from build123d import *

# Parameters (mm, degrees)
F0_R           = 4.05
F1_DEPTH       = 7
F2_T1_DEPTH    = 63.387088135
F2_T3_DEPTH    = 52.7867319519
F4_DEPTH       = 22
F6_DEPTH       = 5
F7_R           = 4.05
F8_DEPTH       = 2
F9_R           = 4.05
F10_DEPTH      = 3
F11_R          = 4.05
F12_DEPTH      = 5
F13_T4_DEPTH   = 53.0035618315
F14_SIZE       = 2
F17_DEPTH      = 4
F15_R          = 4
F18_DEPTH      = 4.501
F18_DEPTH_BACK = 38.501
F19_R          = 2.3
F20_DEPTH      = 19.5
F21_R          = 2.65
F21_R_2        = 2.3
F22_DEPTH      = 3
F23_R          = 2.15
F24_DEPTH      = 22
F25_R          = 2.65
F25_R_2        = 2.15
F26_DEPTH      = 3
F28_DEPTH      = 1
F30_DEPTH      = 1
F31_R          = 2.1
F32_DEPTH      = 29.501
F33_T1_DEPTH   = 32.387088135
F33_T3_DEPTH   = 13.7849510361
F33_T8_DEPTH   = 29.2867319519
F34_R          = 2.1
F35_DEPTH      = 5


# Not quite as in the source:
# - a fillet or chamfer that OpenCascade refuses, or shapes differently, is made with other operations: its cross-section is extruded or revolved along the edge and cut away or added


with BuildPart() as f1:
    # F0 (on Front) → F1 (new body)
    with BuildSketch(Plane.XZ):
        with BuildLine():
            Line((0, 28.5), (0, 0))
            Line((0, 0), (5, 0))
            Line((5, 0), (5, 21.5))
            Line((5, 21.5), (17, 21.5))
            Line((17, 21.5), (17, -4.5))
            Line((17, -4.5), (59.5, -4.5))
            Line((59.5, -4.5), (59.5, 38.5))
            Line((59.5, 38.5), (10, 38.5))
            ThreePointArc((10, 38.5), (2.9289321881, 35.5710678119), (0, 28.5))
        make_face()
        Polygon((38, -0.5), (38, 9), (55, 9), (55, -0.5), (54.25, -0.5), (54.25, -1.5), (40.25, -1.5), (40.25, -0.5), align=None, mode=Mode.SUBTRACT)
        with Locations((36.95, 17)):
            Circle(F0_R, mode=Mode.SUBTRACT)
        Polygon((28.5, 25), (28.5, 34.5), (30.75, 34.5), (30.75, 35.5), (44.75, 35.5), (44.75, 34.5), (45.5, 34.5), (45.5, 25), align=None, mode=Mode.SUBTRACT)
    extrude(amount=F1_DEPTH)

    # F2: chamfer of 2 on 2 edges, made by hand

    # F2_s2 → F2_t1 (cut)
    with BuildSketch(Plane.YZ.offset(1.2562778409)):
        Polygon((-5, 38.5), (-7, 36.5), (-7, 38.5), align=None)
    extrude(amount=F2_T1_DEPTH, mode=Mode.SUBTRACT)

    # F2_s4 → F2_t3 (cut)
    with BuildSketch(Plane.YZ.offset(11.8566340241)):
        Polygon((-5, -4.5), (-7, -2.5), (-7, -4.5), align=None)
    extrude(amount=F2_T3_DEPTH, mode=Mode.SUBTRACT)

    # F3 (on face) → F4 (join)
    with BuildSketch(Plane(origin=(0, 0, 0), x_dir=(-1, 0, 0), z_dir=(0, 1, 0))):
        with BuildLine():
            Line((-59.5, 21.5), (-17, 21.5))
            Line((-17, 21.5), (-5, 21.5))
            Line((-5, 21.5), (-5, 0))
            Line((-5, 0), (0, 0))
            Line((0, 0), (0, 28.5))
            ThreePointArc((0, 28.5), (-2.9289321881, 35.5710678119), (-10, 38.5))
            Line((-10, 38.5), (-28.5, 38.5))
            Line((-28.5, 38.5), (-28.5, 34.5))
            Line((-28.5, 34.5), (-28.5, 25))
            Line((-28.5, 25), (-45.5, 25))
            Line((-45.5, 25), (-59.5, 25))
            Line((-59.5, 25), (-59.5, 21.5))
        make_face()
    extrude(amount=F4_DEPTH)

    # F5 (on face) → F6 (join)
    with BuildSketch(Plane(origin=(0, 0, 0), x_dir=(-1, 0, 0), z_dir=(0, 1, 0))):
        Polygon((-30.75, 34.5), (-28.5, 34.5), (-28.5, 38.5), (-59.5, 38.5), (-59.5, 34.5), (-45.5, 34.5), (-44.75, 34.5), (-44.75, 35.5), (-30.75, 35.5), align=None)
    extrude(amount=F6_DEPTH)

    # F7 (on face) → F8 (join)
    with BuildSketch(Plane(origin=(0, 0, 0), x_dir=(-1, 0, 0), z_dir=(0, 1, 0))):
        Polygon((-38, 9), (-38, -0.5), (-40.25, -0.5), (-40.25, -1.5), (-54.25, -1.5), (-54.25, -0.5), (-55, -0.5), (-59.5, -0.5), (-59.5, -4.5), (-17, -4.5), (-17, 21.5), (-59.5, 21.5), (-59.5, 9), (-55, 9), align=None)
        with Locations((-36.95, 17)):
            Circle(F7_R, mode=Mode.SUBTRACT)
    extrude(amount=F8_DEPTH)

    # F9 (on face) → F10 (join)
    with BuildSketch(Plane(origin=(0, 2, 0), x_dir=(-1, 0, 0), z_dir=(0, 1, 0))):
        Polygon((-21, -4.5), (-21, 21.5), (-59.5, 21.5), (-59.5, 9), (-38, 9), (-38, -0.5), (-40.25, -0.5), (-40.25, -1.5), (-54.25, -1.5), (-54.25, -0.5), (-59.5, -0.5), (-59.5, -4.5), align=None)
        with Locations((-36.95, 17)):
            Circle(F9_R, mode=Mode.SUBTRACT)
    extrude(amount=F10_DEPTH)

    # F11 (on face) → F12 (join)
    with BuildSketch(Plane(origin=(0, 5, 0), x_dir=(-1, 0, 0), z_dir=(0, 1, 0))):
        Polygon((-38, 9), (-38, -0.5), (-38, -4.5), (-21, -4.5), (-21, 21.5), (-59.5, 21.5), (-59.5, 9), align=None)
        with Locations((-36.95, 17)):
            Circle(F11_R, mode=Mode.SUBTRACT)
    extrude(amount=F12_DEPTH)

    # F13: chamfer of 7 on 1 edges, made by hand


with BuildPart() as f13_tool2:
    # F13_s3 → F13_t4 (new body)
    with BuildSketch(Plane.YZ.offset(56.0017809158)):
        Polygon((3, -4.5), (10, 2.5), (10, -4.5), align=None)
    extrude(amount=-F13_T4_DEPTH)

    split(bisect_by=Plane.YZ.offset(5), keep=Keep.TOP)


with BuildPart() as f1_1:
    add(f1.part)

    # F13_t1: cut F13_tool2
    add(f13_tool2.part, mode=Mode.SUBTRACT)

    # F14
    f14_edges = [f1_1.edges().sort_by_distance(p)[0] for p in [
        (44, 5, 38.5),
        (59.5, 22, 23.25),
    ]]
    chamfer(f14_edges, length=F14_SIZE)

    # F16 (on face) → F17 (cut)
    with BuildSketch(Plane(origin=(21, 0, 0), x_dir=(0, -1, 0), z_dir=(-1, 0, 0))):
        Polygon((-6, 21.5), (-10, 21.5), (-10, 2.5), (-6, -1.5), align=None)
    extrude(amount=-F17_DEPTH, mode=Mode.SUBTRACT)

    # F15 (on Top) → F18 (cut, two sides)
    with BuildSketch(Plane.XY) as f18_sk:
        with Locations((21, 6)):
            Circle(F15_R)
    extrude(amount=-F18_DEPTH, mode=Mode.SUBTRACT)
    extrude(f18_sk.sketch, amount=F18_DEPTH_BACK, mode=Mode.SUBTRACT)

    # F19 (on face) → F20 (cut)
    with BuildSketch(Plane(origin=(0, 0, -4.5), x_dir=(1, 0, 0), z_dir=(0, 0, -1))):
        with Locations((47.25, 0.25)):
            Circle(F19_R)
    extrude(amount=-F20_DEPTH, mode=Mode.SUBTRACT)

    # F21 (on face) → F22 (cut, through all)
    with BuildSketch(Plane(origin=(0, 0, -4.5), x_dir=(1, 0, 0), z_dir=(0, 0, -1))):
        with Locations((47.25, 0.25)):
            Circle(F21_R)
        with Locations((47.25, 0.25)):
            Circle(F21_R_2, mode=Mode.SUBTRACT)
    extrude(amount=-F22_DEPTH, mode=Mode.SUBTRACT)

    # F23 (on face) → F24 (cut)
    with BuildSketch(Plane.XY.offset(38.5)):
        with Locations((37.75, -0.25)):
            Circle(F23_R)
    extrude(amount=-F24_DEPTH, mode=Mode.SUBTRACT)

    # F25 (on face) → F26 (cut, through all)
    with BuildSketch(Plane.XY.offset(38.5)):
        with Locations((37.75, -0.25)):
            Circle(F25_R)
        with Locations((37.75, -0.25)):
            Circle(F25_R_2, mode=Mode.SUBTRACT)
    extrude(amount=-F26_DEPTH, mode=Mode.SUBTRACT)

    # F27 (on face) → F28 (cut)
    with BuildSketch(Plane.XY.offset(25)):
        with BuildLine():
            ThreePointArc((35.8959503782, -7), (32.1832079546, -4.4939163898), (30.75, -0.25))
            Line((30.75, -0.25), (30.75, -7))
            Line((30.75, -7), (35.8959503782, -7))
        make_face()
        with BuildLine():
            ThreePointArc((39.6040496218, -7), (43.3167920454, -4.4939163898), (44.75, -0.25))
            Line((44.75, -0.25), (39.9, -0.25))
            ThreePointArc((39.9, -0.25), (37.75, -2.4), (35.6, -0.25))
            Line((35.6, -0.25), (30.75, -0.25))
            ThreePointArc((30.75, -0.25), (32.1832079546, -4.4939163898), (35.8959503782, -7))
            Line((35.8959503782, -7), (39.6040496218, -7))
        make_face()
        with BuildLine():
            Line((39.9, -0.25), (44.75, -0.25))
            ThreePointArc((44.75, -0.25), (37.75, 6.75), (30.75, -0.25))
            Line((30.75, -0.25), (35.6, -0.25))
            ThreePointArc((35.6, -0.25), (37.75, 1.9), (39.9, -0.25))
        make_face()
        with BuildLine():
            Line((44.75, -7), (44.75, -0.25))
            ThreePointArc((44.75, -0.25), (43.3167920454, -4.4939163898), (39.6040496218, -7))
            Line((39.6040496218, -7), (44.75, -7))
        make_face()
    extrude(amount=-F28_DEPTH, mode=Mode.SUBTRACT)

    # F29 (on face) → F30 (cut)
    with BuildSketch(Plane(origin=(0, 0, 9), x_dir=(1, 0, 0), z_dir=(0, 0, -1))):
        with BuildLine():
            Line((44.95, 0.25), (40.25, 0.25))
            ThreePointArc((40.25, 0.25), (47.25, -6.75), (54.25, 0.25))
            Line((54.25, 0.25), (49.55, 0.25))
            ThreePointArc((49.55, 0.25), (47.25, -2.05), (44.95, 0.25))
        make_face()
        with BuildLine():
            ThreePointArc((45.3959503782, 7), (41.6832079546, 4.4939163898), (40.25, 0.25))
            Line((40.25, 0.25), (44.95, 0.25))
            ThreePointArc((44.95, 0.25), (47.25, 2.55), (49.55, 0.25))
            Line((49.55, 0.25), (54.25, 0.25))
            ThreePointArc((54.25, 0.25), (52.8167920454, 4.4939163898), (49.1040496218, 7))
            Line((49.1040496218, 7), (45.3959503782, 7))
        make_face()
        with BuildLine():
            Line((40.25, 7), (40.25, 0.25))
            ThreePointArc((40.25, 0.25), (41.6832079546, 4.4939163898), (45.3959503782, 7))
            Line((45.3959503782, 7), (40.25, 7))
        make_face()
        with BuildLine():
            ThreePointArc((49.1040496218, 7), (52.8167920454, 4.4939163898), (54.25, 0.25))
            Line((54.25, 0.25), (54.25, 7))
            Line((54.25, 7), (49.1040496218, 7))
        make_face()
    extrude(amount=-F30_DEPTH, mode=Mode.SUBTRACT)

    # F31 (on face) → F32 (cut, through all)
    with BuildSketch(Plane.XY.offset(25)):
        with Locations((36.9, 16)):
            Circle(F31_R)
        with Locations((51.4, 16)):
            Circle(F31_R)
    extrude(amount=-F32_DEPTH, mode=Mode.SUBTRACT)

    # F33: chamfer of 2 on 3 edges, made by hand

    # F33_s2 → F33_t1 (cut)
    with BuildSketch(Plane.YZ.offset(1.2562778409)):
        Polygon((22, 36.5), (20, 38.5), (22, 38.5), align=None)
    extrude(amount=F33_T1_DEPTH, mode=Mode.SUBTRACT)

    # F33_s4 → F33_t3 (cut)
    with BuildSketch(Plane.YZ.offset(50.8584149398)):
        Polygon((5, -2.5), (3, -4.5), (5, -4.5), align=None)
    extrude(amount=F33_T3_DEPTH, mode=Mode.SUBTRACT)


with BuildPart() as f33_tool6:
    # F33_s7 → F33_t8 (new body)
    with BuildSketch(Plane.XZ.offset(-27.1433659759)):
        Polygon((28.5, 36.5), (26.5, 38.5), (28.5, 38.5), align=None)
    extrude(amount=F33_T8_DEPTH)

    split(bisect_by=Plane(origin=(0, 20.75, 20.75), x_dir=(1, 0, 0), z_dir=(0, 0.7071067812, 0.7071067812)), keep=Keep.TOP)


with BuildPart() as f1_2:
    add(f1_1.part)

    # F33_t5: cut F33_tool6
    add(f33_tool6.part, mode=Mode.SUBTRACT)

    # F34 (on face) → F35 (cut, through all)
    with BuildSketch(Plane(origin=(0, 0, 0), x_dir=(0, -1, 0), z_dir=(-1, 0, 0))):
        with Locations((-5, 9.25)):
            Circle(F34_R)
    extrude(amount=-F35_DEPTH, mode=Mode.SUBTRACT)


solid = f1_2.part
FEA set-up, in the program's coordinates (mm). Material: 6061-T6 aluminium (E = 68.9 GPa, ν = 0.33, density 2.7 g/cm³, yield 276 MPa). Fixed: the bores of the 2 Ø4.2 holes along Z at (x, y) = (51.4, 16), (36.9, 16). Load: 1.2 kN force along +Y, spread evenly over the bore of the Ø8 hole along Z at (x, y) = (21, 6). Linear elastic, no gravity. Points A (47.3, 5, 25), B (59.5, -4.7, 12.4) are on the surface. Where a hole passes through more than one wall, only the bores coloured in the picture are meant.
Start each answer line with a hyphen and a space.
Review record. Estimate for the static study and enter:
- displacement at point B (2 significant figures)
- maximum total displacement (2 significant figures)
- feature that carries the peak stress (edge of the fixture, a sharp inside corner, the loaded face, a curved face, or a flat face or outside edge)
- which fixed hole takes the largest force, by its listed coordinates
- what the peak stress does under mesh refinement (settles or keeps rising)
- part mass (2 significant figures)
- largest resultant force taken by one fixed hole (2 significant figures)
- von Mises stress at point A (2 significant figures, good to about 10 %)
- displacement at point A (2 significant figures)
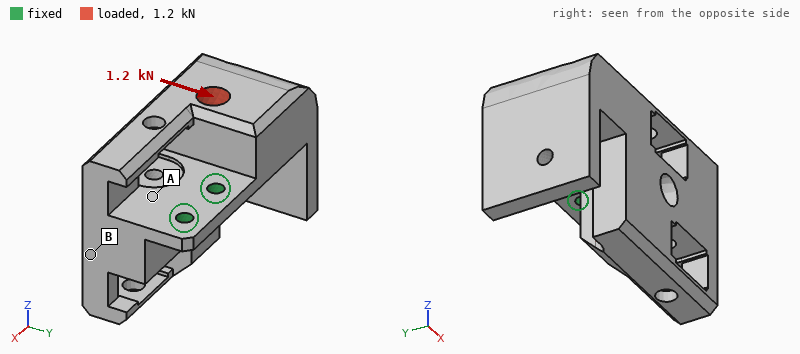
- 33 µm
- 62 µm
- edge of the fixture
- (36.9, 16)
- keeps rising
- 87 g
- 2.1 kN
- 16 MPa
- 11 µm
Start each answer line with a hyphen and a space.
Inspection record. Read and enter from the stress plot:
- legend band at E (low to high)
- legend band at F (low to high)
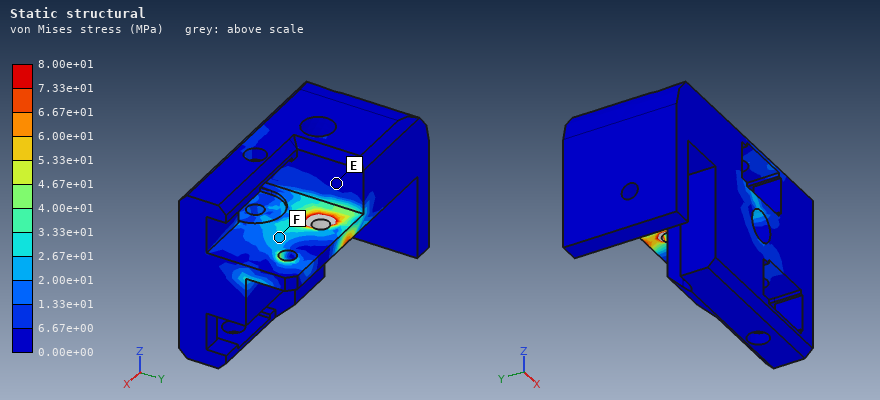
- 0.00e+00 to 6.67e+00 MPa
- 2.00e+01 to 2.67e+01 MPa
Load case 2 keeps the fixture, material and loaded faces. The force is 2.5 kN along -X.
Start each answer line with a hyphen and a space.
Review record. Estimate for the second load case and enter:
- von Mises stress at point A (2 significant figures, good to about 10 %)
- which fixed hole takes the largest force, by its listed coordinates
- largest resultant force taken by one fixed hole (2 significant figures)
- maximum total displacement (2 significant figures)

- 37 MPa
- (36.9, 16)
- 2.1 kN
- 87 µm
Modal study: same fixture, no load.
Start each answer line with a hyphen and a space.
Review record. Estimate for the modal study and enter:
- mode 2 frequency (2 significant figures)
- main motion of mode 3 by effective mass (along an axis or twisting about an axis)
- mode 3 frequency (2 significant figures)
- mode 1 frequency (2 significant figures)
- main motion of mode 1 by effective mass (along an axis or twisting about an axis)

- 2100 Hz
- along Y
- 3200 Hz
- 1200 Hz
- along Z
